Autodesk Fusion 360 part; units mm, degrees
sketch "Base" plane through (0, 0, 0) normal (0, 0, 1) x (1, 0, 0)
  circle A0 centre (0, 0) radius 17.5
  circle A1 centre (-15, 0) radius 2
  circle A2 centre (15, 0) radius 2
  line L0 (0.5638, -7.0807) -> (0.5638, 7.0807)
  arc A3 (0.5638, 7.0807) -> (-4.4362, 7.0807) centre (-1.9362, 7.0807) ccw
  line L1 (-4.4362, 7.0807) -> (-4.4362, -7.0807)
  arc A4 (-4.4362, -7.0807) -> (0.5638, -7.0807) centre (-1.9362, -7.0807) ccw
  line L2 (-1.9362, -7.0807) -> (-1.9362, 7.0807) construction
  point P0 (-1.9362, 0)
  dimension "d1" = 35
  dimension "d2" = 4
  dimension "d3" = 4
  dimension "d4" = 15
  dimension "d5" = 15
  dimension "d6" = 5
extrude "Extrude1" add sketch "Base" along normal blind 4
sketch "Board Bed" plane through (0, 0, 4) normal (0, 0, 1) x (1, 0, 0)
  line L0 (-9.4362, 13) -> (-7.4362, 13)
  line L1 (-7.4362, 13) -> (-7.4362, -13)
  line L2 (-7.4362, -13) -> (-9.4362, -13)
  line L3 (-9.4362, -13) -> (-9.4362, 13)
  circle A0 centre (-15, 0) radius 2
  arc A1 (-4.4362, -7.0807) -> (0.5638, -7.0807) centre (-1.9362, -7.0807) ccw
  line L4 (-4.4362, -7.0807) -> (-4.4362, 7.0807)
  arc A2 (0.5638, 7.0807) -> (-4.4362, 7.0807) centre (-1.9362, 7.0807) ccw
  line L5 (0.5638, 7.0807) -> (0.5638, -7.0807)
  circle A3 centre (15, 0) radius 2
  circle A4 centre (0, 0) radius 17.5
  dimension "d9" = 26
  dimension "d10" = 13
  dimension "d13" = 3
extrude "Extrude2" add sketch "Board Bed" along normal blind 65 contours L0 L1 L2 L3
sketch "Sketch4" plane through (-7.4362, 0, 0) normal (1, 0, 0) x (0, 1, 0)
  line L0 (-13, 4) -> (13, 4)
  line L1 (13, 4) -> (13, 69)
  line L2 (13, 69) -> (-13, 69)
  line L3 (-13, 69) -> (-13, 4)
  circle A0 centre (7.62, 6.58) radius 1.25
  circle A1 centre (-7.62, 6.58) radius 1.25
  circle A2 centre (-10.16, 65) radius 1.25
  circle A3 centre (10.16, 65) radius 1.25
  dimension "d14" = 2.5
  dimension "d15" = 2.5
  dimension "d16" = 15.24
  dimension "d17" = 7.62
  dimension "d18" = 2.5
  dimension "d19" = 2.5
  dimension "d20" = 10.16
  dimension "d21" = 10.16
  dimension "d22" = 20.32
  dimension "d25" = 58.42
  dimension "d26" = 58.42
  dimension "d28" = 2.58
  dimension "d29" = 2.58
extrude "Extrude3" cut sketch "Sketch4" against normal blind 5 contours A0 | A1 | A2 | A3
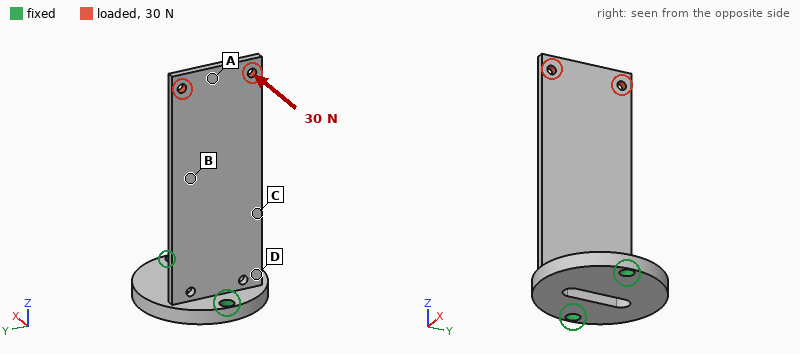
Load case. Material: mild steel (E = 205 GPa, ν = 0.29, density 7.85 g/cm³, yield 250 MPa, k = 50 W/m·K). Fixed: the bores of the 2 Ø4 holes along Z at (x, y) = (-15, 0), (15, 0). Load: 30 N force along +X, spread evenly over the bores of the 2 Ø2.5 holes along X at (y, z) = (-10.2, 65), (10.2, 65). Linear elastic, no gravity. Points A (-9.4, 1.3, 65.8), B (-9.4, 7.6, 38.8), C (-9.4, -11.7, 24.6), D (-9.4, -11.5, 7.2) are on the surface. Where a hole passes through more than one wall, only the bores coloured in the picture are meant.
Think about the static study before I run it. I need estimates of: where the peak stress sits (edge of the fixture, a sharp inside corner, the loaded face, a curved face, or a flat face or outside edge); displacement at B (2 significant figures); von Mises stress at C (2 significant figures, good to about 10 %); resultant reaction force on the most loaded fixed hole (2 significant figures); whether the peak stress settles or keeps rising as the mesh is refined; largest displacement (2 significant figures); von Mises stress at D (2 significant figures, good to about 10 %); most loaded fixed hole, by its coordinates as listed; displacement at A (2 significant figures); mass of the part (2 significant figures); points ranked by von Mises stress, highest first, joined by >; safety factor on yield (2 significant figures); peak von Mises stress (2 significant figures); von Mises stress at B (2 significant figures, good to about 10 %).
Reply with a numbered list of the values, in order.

1. a curved face
2. 0.28 mm
3. 71 MPa
4. 68 N
5. settles
6. 0.75 mm
7. 110 MPa
8. (-15, 0)
9. 0.70 mm
10. 53 g
11. D > C > B > A
12. 1.2
13. 210 MPa
14. 45 MPa
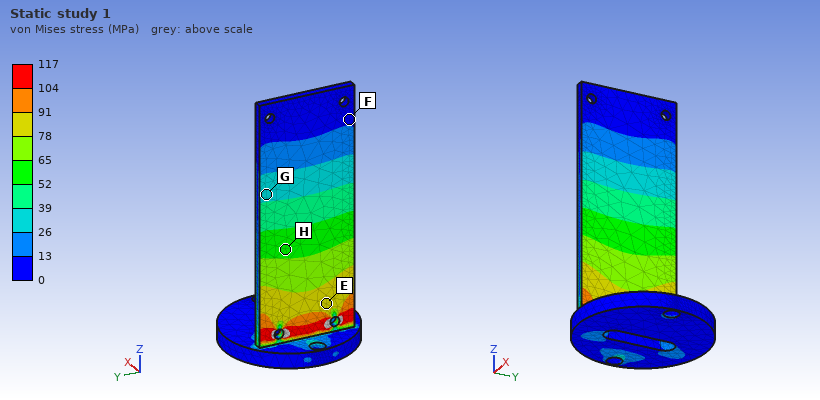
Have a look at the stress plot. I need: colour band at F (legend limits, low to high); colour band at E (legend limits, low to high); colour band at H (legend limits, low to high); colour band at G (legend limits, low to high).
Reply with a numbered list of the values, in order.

1. 0 to 13 MPa
2. 78 to 91 MPa
3. 52 to 65 MPa
4. 26 to 39 MPa
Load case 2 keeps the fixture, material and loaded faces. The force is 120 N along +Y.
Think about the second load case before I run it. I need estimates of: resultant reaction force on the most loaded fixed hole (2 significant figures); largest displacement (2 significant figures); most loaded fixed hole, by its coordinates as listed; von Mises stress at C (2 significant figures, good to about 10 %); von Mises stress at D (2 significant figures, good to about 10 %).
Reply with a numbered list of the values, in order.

1. 100 N
2. 89 µm
3. (-15, 0)
4. 20 MPa
5. 29 MPa
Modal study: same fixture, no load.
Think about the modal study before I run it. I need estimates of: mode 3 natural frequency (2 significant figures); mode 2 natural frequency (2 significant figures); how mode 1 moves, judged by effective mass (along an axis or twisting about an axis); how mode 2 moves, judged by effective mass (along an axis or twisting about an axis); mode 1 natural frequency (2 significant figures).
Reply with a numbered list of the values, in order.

1. 2000 Hz
2. 1900 Hz
3. along X
4. along Y
5. 380 Hz
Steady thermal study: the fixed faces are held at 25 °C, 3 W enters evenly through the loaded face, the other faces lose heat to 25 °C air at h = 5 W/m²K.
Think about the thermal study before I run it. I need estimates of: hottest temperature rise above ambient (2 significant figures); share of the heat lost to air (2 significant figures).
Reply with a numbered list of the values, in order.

1. 70 K
2. 23 %
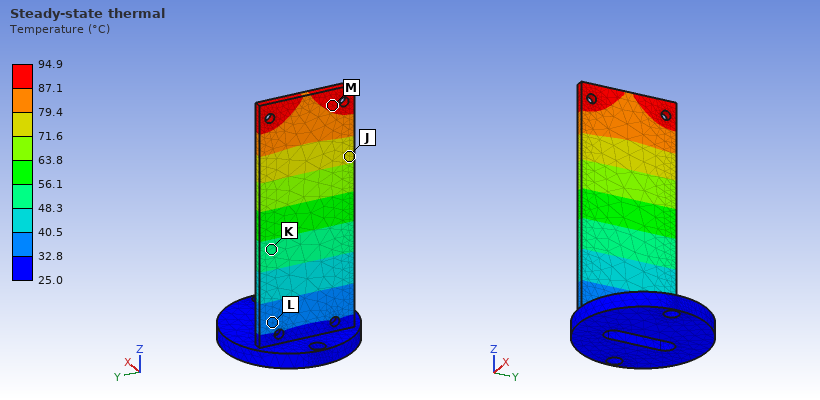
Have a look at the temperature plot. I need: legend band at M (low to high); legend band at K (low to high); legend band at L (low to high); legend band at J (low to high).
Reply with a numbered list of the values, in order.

1. 87.1 to 94.9 °C
2. 48.3 to 56.1 °C
3. 32.8 to 40.5 °C
4. 71.6 to 79.4 °C
